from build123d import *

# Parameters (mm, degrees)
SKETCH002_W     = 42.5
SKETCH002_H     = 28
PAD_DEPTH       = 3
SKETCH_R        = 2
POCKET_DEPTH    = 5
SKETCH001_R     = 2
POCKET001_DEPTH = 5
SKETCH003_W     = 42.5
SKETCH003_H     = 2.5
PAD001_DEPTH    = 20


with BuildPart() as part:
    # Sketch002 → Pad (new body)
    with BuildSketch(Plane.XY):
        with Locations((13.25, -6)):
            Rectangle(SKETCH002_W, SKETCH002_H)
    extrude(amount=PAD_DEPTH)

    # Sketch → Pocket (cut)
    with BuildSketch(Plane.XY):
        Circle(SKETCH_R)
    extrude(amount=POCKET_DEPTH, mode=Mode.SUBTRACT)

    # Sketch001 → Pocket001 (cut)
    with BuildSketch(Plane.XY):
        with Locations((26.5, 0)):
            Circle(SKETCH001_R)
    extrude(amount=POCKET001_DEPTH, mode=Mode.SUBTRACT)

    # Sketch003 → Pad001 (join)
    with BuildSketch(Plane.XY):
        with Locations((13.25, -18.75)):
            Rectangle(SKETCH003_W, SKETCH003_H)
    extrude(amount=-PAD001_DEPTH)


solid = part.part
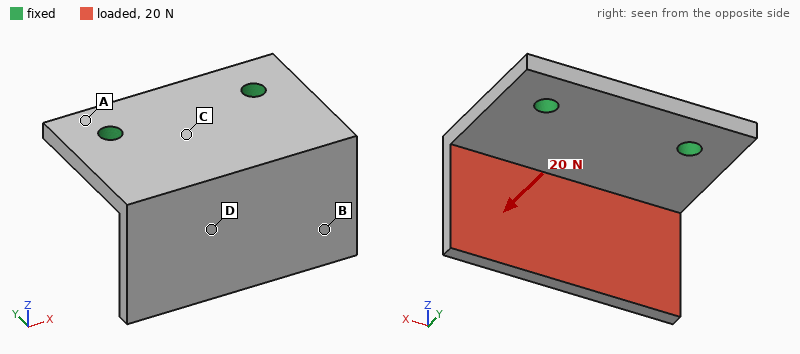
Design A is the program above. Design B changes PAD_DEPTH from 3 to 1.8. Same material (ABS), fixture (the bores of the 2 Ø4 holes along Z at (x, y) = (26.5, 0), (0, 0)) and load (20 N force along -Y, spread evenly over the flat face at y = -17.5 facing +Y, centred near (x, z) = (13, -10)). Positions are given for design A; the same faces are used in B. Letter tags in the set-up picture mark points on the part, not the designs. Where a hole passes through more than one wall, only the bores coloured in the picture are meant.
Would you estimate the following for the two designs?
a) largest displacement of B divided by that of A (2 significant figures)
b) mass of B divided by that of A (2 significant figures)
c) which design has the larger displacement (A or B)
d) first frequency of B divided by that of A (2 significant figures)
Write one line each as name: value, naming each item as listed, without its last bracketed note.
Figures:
largest displacement of B divided by that of A: 3.2
mass of B divided by that of A: 0.75
which design has the larger displacement: B
first frequency of B divided by that of A: 0.52
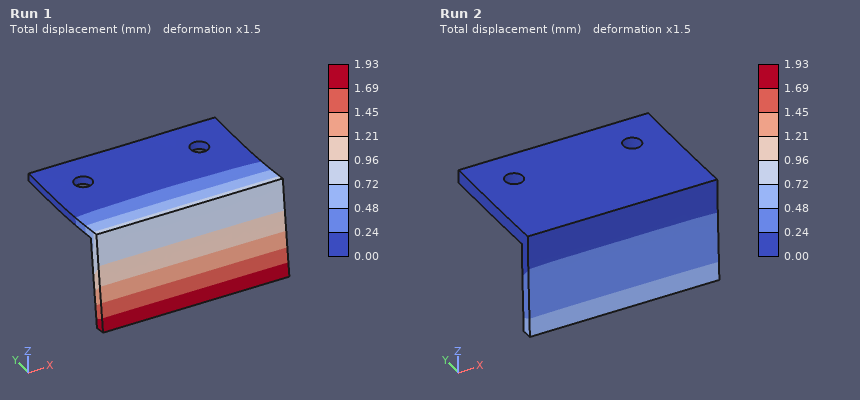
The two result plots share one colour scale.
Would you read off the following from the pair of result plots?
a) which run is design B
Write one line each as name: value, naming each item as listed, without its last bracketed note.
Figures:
which run is design B: Run 1
